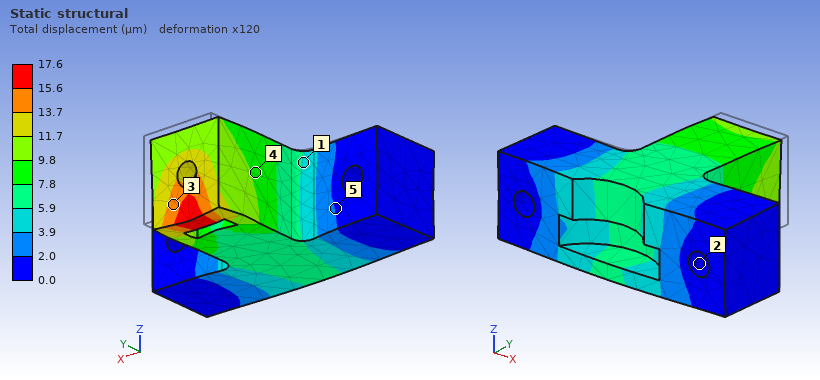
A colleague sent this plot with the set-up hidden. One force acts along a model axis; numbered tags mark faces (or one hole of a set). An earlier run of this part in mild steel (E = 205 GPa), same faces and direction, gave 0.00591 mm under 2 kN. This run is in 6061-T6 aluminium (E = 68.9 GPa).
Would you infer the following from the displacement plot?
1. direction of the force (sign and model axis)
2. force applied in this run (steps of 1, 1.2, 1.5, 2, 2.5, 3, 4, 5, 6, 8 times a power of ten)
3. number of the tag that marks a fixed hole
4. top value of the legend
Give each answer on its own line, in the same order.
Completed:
-Y
2 kN
2
17.6 µm
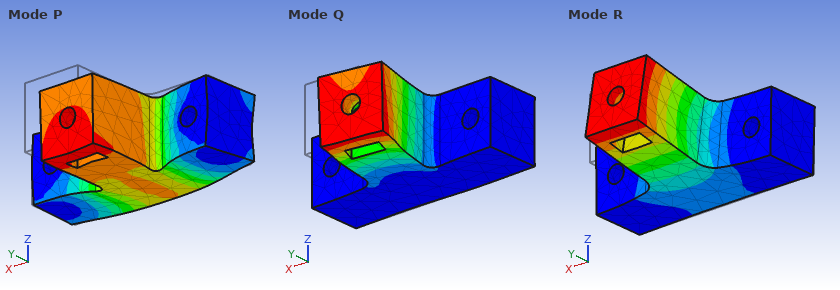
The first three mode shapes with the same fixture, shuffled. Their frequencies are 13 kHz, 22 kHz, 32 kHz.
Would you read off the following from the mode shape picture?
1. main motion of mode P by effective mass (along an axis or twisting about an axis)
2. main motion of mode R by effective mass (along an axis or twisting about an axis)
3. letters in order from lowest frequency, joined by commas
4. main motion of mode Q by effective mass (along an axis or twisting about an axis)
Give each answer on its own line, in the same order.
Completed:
along Y
along Z
R, Q, P
along X
